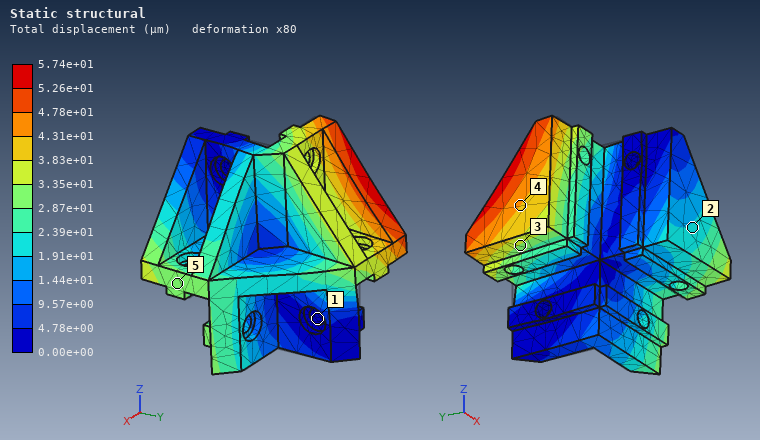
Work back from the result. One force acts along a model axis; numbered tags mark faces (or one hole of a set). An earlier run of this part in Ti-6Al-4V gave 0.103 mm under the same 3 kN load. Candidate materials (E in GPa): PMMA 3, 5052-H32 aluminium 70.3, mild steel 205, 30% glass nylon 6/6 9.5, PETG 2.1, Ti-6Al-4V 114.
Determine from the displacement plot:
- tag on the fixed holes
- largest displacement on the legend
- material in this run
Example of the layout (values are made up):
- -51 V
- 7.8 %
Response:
- 1
- 5.74e+01 µm
- mild steel
